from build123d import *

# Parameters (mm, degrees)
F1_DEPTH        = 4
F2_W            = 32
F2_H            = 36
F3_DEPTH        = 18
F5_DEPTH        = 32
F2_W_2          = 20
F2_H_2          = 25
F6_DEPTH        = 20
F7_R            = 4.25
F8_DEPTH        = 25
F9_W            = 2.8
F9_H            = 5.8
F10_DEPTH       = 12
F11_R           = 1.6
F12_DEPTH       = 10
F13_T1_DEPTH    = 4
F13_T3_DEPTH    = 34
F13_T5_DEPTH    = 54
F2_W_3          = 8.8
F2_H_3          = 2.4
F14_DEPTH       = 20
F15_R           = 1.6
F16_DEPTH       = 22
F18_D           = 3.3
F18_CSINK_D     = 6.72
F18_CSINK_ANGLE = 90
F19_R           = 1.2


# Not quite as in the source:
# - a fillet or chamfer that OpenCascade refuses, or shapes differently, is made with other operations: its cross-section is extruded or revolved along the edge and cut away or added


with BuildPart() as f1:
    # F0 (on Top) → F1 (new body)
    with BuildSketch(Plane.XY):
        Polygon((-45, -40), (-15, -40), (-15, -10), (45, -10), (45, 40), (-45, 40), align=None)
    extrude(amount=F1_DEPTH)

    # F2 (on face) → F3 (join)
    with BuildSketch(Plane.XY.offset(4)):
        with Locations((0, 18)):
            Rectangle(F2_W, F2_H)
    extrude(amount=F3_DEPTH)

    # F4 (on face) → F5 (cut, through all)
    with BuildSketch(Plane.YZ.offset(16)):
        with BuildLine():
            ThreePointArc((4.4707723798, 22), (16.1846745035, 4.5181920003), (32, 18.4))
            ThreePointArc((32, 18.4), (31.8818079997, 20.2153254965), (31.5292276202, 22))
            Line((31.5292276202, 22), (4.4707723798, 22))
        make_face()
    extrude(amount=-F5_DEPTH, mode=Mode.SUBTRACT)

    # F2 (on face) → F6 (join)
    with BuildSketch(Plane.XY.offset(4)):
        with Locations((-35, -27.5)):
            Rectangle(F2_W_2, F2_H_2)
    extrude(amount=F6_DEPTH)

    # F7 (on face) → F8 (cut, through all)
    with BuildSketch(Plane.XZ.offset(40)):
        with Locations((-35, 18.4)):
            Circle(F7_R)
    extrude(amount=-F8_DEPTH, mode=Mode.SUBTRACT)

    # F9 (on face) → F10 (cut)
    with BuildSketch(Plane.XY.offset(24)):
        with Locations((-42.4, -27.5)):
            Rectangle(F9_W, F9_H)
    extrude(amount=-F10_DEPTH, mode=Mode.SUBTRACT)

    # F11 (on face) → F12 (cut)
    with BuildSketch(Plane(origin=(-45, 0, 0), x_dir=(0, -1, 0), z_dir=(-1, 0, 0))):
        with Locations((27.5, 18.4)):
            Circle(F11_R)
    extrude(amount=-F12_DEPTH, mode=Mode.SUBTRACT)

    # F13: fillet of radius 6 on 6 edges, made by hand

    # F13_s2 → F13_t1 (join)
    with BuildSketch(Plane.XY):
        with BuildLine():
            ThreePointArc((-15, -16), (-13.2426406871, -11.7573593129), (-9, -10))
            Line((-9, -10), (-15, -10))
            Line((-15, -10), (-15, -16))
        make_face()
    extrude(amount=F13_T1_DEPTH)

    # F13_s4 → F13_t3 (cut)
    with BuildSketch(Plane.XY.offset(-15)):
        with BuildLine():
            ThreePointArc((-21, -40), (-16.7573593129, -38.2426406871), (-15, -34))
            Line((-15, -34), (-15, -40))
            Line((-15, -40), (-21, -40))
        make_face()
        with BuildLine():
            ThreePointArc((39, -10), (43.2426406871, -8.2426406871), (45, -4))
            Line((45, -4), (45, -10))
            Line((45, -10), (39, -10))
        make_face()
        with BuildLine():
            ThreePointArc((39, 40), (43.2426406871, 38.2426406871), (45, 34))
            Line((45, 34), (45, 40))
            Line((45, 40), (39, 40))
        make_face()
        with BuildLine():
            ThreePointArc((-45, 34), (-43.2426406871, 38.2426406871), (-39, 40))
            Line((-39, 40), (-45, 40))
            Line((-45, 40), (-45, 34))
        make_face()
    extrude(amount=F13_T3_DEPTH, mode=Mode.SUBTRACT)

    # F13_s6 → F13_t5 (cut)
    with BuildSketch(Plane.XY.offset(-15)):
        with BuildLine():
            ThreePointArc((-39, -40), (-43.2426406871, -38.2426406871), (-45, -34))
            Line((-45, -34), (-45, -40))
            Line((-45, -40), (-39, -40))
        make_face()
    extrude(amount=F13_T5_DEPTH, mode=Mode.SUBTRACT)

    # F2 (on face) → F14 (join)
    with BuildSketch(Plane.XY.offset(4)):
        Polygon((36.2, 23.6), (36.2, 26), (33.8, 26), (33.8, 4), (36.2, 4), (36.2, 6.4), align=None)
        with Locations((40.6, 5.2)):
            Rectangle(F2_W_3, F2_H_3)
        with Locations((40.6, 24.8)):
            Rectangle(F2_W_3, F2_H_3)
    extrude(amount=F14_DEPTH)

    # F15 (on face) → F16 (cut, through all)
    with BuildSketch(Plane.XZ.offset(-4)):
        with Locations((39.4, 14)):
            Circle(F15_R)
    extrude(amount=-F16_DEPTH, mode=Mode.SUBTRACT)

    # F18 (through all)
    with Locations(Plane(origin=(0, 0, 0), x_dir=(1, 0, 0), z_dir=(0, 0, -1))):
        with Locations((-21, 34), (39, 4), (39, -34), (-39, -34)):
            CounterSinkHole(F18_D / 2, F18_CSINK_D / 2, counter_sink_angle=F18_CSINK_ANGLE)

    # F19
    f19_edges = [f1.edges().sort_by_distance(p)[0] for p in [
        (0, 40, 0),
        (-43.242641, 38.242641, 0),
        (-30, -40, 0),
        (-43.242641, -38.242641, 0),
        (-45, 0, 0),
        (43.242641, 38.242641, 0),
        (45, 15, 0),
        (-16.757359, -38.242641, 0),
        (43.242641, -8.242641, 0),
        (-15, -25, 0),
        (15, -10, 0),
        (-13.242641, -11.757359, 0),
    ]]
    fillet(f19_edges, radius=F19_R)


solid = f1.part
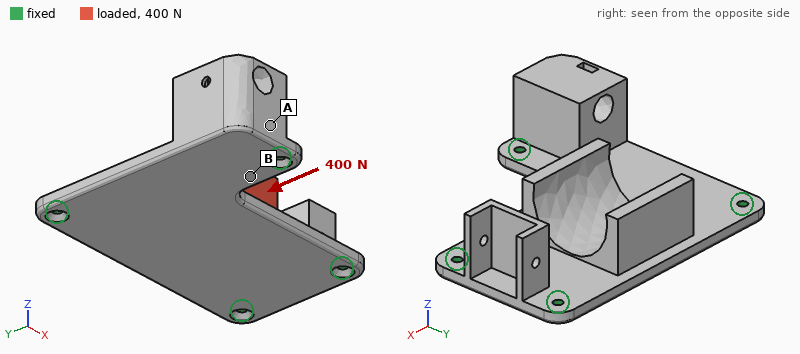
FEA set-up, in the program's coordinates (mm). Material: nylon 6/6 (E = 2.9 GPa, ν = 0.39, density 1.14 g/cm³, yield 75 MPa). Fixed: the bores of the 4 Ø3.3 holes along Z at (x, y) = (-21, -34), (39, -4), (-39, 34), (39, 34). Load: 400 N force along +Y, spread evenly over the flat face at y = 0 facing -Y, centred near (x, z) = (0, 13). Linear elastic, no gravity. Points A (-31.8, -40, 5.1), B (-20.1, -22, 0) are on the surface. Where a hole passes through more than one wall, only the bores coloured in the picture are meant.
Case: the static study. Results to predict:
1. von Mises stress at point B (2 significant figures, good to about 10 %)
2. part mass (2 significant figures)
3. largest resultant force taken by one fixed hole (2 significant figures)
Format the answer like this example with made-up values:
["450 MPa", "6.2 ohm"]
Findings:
["5.9 MPa", "44 g", "140 N"]
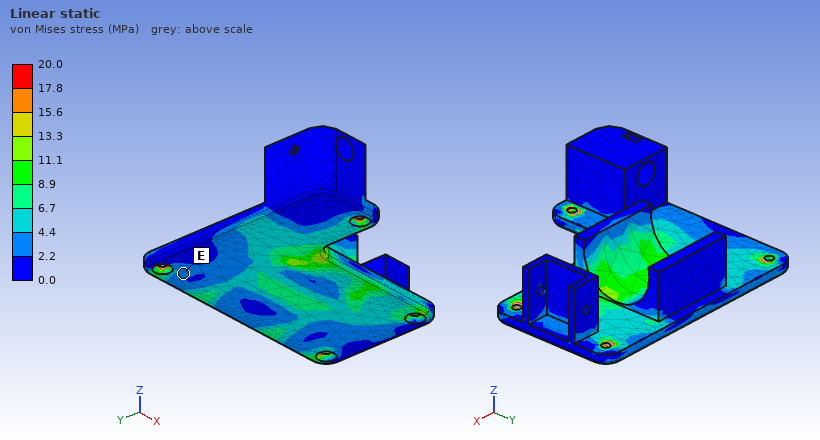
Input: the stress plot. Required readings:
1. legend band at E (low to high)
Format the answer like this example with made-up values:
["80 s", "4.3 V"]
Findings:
["2.2 to 4.4 MPa"]
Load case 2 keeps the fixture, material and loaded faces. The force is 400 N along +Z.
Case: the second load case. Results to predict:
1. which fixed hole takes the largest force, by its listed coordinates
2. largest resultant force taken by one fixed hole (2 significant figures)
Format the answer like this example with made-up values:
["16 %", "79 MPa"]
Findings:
["(39, -4)", "170 N"]
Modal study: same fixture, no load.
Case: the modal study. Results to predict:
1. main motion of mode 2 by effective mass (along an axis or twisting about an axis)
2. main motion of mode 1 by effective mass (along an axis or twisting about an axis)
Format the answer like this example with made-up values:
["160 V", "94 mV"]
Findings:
["along Z", "along Z"]
